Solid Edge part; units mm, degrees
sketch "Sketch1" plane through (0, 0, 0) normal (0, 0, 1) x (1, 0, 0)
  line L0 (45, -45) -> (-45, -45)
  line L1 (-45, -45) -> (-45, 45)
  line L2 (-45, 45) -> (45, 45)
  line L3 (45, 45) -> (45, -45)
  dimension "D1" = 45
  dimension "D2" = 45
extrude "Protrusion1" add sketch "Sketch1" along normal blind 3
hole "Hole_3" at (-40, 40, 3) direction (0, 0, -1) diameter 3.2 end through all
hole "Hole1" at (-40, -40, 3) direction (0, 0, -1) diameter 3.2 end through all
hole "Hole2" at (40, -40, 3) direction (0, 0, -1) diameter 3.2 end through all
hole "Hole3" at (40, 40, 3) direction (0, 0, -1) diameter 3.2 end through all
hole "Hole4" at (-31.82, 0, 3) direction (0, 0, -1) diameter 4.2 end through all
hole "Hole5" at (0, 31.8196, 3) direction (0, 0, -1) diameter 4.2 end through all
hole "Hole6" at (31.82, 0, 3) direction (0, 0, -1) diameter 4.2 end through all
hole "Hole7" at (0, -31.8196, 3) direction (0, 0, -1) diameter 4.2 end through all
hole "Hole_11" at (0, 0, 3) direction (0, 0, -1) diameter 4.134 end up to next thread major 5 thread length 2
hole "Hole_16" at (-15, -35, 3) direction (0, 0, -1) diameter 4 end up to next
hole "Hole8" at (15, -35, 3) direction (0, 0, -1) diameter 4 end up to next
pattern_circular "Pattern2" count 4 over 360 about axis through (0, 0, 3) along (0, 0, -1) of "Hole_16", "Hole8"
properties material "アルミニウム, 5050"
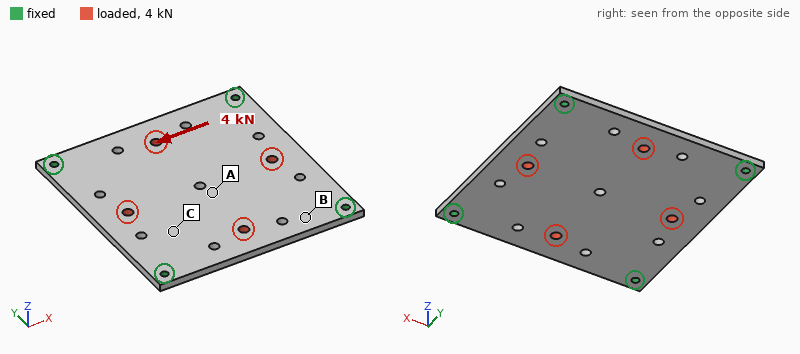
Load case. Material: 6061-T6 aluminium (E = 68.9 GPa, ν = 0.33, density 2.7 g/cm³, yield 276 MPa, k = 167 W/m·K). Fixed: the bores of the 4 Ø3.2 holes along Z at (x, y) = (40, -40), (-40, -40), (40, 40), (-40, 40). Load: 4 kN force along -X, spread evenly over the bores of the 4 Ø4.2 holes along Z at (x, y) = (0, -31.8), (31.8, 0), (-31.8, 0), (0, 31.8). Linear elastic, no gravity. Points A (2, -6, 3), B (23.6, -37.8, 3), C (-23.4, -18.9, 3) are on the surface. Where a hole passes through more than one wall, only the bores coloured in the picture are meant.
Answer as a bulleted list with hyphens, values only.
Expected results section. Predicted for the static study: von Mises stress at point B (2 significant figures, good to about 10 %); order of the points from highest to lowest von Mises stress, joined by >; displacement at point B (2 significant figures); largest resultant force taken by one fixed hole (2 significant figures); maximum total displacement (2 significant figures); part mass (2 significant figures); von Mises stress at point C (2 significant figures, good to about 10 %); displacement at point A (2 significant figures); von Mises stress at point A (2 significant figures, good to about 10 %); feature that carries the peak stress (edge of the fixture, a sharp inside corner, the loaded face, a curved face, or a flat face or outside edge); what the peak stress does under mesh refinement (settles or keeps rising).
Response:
- 15 MPa
- B > C > A
- 5.9 µm
- 1.1 kN
- 17 µm
- 64 g
- 8.9 MPa
- 12 µm
- 4.1 MPa
- edge of the fixture
- keeps rising
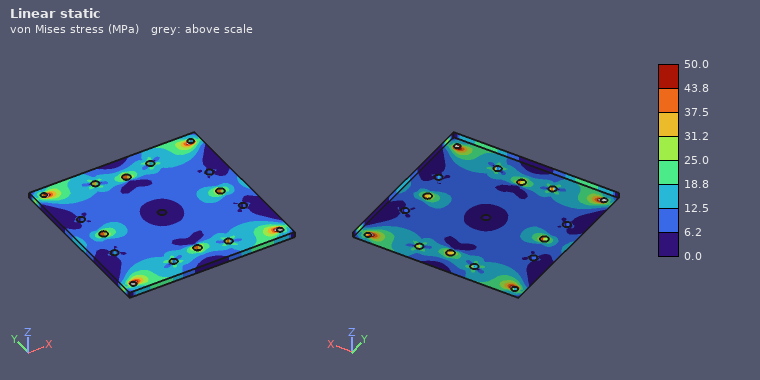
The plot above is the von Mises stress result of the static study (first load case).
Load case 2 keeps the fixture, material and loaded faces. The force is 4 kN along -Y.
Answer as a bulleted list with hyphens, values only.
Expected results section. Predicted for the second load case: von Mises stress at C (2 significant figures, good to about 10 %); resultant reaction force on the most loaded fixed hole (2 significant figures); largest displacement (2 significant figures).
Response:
- 9.8 MPa
- 1.1 kN
- 17 µm
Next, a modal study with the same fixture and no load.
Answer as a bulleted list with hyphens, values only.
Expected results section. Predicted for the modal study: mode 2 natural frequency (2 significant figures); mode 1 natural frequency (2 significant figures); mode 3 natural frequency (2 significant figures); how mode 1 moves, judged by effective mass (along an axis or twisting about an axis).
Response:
- 2600 Hz
- 1500 Hz
- 2600 Hz
- along Z
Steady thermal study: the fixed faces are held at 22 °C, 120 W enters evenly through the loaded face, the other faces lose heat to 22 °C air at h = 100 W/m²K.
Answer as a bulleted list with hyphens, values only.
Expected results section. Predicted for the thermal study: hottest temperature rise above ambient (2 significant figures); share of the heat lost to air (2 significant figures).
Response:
- 56 K
- 46 %
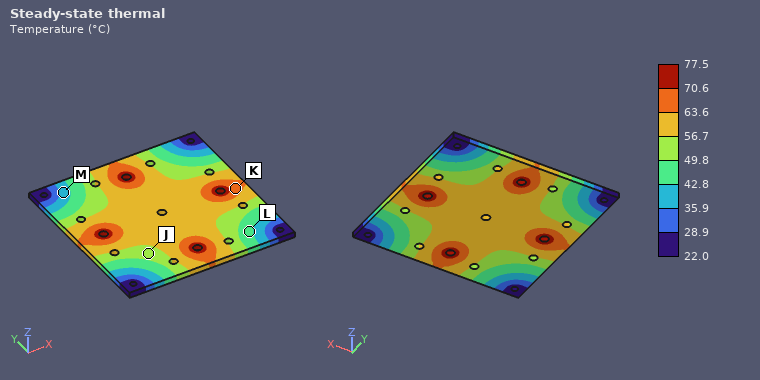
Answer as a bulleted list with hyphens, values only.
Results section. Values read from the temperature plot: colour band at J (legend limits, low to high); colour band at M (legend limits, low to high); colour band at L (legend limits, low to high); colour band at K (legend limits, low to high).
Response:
- 49.8 to 56.7 °C
- 35.9 to 42.8 °C
- 42.8 to 49.8 °C
- 63.6 to 70.6 °C
